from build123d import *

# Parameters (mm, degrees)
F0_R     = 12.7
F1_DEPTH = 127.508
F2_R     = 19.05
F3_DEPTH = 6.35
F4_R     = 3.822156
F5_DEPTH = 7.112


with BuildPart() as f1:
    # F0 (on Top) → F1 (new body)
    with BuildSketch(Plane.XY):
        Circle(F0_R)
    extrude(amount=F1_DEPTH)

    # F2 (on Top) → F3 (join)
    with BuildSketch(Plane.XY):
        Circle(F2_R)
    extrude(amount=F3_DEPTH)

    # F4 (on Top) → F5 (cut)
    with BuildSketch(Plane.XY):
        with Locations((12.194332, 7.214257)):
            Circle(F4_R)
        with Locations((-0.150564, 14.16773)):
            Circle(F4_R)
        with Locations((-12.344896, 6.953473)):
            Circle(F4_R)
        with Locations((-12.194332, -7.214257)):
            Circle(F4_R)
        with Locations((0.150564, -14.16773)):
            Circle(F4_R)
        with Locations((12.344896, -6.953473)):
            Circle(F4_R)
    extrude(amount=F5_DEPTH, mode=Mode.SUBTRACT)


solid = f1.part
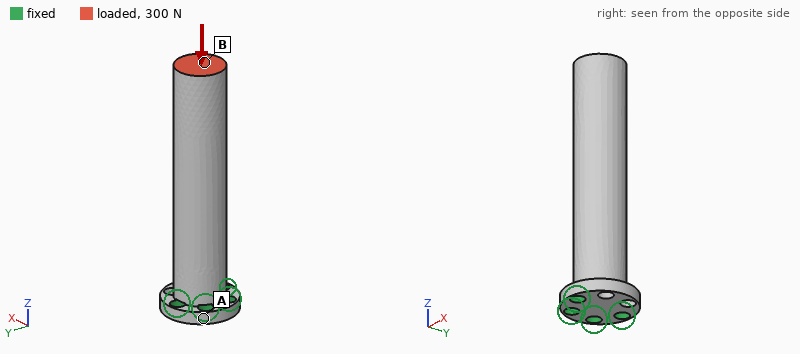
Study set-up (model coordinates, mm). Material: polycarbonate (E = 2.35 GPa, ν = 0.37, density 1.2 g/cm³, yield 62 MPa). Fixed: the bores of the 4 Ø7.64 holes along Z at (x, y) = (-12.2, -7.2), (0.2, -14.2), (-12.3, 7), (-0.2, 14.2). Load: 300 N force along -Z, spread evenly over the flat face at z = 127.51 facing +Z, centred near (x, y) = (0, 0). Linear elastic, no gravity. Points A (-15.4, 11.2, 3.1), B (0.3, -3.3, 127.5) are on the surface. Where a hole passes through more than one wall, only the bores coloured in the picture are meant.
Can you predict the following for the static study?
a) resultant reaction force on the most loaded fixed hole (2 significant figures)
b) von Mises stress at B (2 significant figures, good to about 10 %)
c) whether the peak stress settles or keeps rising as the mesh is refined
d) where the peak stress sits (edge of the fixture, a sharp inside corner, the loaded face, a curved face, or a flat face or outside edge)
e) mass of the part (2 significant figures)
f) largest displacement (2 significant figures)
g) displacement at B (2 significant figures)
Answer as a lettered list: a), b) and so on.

a) 120 N
b) 0.59 MPa
c) keeps rising
d) edge of the fixture
e) 80 g
f) 73 µm
g) 69 µm
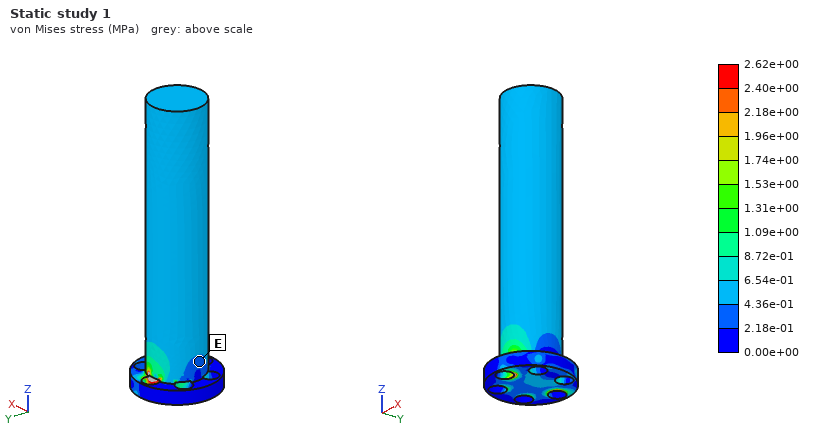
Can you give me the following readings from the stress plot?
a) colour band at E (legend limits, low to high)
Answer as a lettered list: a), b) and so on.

a) 2.18e-01 to 4.36e-01 MPa
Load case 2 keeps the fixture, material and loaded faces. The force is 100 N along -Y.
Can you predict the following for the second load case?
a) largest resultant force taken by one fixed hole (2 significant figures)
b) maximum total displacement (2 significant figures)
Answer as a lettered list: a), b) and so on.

a) 440 N
b) 1.4 mm
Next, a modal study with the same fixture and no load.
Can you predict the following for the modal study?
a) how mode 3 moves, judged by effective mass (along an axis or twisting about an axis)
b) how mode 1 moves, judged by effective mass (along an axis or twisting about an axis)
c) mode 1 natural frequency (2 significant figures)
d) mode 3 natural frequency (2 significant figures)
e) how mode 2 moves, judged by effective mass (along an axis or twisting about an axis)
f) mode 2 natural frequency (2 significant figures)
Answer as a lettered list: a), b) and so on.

a) along X
b) along X
c) 270 Hz
d) 1600 Hz
e) along Y
f) 310 Hz
